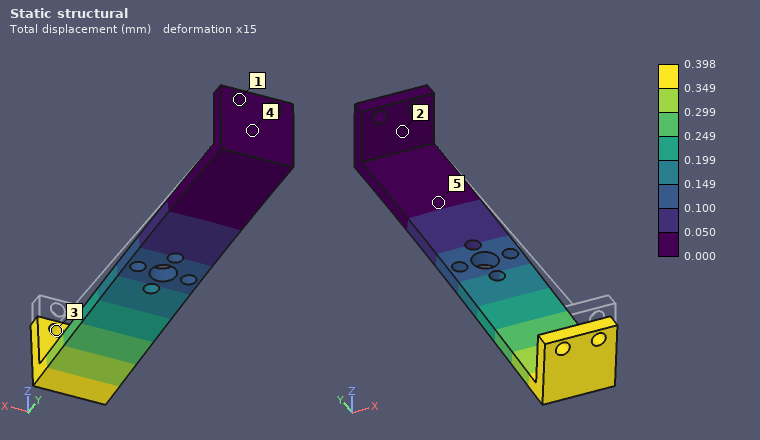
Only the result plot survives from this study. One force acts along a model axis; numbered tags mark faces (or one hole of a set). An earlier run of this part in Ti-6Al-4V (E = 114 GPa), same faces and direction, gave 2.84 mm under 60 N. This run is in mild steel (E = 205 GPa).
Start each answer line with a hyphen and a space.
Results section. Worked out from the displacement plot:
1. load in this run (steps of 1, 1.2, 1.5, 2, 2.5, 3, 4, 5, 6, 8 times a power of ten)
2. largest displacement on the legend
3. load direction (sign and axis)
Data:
- 15 N
- 0.398 mm
- -Z
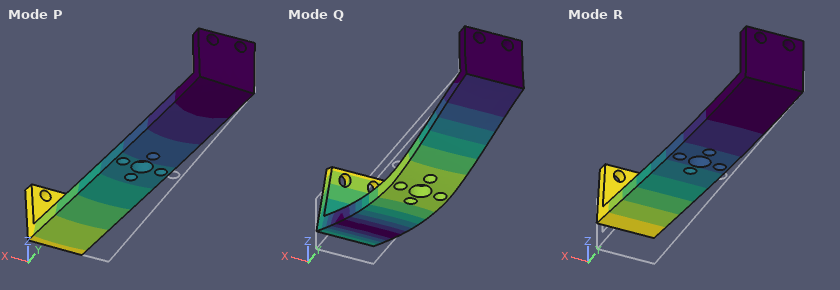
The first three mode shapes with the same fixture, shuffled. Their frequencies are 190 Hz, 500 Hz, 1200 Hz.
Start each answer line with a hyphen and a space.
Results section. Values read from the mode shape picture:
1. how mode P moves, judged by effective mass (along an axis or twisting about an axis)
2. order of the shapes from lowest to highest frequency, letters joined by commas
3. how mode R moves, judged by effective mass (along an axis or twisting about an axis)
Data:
- along X
- R, P, Q
- along Z
